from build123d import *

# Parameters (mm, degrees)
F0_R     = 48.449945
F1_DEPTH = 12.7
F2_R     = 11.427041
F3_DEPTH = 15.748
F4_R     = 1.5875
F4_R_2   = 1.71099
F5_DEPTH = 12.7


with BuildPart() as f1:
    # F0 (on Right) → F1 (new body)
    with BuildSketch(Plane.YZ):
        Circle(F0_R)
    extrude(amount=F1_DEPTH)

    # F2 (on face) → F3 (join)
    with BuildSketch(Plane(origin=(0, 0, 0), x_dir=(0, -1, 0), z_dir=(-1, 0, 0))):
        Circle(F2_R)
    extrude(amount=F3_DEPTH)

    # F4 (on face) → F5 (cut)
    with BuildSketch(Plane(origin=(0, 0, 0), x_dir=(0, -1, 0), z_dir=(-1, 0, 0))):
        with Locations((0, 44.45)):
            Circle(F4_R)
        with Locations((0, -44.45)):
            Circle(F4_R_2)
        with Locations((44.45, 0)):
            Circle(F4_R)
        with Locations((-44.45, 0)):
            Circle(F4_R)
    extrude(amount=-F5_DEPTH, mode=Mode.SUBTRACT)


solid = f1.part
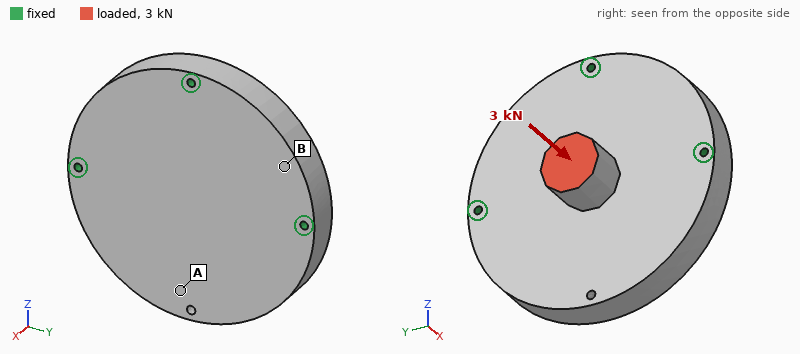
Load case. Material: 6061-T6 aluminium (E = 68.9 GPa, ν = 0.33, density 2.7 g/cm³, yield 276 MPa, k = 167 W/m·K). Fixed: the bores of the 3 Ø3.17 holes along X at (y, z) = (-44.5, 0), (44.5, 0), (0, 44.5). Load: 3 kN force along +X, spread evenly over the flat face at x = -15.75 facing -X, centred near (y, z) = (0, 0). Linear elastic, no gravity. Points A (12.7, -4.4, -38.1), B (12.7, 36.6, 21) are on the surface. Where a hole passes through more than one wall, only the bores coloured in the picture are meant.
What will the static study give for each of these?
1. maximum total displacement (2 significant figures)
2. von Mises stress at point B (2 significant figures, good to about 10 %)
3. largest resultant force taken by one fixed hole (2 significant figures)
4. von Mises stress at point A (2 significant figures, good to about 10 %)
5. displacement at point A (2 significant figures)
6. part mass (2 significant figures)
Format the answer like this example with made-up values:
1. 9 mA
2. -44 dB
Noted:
1. 43 µm
2. 4.4 MPa
3. 1.2 kN
4. 9.6 MPa
5. 37 µm
6. 270 g
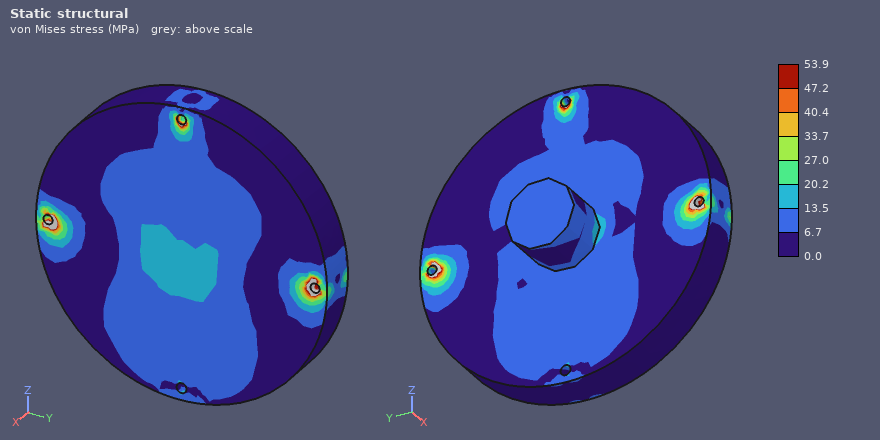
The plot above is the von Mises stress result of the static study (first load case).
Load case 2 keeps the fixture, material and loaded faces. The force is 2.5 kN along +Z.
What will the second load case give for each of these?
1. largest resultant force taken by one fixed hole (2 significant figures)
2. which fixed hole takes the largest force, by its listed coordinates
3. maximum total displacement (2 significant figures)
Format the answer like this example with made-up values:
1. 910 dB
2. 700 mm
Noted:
1. 1.4 kN
2. (0, 44.5)
3. 43 µm
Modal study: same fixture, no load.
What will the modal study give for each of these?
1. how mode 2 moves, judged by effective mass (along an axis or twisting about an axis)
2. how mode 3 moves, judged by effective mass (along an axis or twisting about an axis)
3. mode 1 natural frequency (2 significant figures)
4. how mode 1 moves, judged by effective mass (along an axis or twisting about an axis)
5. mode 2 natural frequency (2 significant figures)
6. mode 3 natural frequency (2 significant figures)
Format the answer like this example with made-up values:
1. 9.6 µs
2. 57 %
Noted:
1. along X
2. twisting about Z
3. 3200 Hz
4. along X
5. 8400 Hz
6. 8800 Hz
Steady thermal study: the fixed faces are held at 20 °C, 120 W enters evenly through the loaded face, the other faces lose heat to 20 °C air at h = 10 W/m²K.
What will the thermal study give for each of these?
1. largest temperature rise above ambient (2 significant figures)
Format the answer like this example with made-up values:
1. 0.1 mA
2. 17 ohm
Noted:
1. 56 K
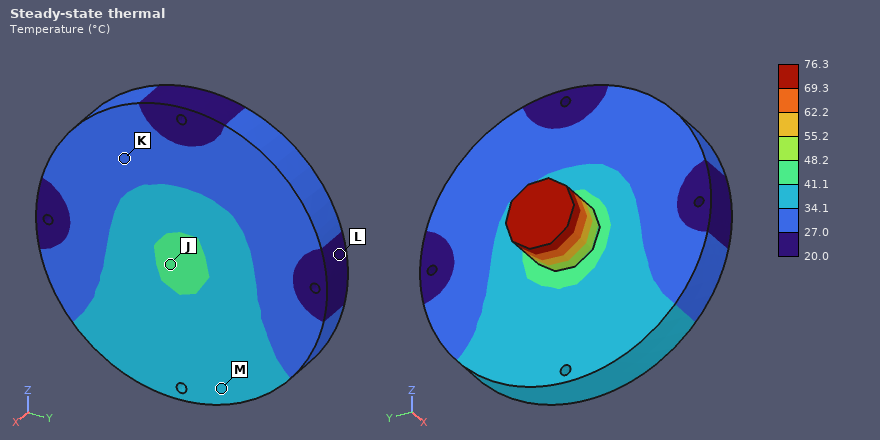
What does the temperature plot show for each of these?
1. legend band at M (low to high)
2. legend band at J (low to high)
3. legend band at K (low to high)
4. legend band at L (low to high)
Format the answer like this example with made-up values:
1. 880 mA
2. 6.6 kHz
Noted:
1. 34.1 to 41.1 °C
2. 41.1 to 48.2 °C
3. 27.0 to 34.1 °C
4. 20.0 to 27.0 °C
